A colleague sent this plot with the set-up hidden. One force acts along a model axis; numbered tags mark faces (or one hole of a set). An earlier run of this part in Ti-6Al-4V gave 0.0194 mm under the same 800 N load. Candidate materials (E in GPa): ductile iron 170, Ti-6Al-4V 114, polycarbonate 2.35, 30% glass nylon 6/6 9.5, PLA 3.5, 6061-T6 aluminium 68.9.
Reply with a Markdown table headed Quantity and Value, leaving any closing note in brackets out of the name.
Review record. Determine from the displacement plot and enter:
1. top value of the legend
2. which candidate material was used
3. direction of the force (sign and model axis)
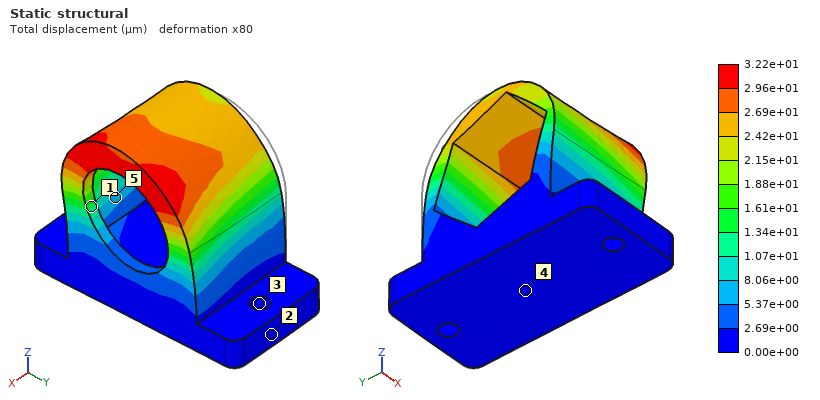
| Quantity | Value |
|---|---|
| top value of the legend | 3.22e+01 µm |
| which candidate material was used | 6061-T6 aluminium |
| direction of the force | -Y |
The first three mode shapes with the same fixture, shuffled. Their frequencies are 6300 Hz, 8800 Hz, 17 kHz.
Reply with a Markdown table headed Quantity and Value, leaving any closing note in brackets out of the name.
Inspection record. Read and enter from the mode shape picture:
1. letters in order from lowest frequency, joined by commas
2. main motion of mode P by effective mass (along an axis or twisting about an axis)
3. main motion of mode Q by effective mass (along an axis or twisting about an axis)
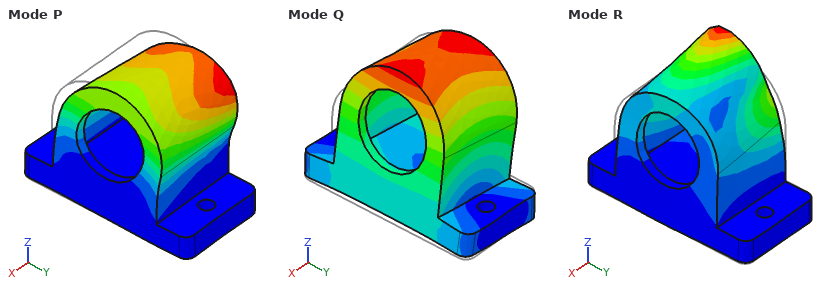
| Quantity | Value |
|---|---|
| letters in order from lowest frequency, joined by commas | Q, P, R |
| main motion of mode P by effective mass | along Y |
| main motion of mode Q by effective mass | along X |
